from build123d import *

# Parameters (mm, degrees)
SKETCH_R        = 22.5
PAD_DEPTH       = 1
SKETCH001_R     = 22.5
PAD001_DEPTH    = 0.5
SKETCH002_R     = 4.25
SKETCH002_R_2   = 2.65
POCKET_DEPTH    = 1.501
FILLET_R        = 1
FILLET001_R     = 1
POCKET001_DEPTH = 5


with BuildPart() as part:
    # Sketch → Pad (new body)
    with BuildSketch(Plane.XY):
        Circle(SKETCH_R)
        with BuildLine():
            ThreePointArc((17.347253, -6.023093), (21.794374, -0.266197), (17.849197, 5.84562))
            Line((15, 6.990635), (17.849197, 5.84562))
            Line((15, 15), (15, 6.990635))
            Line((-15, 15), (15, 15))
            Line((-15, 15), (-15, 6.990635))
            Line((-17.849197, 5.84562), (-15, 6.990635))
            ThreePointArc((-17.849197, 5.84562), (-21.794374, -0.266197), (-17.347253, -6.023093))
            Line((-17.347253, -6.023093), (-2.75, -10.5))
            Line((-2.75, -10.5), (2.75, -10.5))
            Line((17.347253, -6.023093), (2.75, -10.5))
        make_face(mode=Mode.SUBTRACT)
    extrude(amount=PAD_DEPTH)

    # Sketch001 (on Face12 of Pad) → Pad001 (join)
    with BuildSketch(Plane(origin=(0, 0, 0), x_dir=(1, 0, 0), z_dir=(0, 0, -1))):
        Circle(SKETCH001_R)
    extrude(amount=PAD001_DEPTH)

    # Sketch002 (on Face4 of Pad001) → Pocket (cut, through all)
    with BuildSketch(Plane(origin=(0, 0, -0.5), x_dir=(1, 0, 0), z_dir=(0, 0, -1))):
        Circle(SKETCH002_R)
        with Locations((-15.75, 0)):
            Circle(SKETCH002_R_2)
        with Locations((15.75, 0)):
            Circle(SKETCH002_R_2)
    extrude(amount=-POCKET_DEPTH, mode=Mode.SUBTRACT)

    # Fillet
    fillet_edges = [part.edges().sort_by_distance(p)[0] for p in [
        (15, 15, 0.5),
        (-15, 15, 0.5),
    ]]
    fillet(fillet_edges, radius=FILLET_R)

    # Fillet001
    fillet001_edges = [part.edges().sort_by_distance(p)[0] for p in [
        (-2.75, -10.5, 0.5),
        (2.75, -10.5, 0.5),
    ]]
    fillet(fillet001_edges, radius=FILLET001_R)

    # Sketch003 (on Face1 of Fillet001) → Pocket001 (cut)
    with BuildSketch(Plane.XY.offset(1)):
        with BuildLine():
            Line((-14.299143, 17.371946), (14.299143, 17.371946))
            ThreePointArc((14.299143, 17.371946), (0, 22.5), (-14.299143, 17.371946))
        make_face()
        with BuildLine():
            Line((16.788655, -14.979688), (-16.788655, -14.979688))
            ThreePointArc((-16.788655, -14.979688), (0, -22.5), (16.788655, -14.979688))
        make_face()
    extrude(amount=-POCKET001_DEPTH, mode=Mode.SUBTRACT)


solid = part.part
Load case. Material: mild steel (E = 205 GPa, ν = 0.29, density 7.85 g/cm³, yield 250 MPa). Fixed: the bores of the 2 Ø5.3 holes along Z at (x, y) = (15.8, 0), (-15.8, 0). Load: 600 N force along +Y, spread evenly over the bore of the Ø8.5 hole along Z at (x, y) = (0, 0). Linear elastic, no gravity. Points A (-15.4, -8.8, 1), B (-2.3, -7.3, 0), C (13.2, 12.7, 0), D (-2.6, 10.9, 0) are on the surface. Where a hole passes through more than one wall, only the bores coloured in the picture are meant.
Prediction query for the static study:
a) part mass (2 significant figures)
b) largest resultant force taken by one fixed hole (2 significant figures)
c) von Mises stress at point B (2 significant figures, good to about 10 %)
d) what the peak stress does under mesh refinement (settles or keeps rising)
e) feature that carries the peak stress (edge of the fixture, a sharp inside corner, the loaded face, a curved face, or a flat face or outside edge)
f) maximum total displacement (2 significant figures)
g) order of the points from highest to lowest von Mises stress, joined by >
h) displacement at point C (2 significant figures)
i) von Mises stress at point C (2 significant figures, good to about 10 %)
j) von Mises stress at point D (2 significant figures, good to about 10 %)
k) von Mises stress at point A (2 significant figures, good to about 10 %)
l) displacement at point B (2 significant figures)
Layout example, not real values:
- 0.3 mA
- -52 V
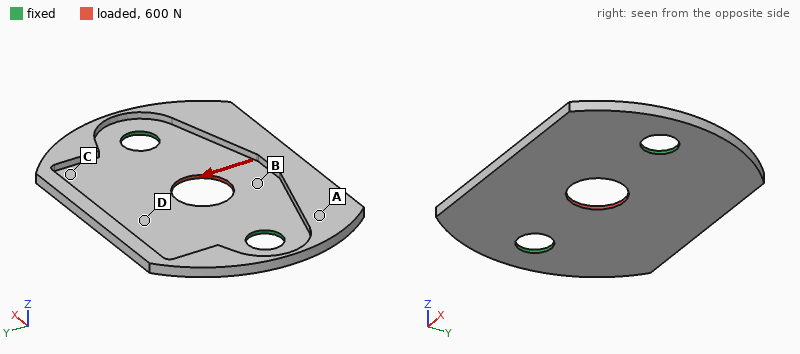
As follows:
- 8.4 g
- 300 N
- 42 MPa
- keeps rising
- edge of the fixture
- 10 µm
- B > D > C > A
- 2.1 µm
- 20 MPa
- 30 MPa
- 8.2 MPa
- 9.8 µm
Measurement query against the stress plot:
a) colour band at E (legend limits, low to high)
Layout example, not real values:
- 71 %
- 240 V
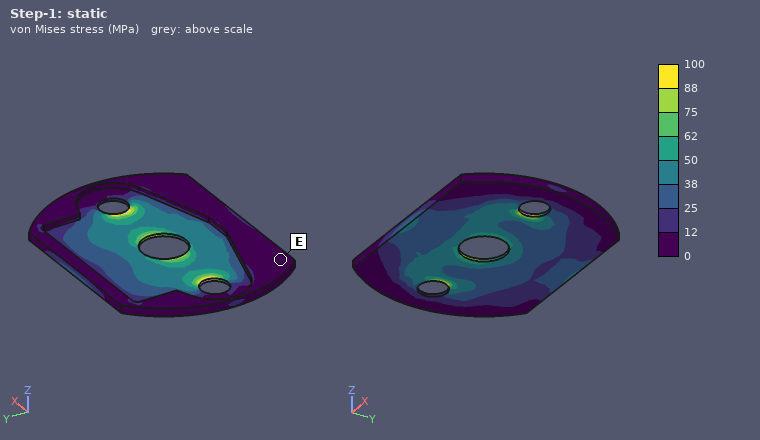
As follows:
- 0 to 12 MPa
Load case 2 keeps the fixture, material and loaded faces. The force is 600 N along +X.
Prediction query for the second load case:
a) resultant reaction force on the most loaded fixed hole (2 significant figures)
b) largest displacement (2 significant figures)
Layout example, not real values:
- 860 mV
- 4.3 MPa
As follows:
- 300 N
- 3.5 µm
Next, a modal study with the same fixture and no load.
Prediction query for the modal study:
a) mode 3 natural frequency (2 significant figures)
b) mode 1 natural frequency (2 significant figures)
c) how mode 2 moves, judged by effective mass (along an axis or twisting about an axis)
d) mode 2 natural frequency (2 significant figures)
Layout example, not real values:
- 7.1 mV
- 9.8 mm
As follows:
- 3500 Hz
- 1800 Hz
- along Z
- 2100 Hz
